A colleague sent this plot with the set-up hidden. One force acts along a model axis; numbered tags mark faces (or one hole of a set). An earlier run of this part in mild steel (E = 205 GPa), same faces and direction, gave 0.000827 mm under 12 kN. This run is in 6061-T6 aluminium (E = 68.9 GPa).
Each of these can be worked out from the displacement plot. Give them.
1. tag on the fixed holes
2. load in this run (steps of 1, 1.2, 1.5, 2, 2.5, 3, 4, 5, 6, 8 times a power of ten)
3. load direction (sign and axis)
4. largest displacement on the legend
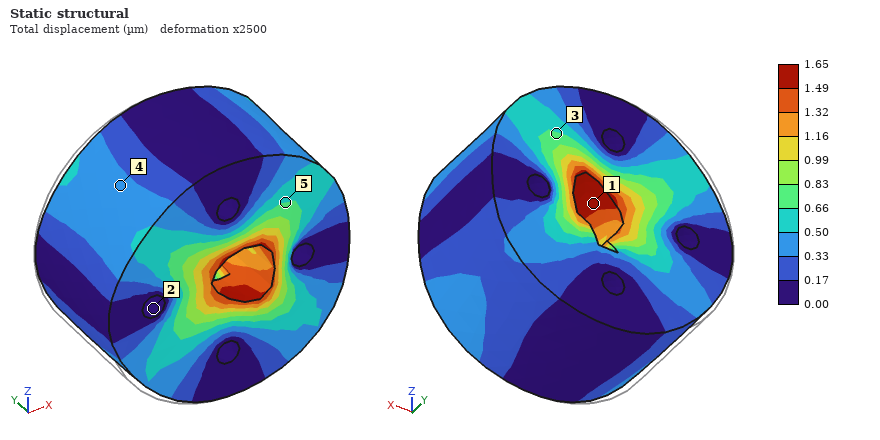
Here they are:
2
8 kN
+X
1.65 µm
